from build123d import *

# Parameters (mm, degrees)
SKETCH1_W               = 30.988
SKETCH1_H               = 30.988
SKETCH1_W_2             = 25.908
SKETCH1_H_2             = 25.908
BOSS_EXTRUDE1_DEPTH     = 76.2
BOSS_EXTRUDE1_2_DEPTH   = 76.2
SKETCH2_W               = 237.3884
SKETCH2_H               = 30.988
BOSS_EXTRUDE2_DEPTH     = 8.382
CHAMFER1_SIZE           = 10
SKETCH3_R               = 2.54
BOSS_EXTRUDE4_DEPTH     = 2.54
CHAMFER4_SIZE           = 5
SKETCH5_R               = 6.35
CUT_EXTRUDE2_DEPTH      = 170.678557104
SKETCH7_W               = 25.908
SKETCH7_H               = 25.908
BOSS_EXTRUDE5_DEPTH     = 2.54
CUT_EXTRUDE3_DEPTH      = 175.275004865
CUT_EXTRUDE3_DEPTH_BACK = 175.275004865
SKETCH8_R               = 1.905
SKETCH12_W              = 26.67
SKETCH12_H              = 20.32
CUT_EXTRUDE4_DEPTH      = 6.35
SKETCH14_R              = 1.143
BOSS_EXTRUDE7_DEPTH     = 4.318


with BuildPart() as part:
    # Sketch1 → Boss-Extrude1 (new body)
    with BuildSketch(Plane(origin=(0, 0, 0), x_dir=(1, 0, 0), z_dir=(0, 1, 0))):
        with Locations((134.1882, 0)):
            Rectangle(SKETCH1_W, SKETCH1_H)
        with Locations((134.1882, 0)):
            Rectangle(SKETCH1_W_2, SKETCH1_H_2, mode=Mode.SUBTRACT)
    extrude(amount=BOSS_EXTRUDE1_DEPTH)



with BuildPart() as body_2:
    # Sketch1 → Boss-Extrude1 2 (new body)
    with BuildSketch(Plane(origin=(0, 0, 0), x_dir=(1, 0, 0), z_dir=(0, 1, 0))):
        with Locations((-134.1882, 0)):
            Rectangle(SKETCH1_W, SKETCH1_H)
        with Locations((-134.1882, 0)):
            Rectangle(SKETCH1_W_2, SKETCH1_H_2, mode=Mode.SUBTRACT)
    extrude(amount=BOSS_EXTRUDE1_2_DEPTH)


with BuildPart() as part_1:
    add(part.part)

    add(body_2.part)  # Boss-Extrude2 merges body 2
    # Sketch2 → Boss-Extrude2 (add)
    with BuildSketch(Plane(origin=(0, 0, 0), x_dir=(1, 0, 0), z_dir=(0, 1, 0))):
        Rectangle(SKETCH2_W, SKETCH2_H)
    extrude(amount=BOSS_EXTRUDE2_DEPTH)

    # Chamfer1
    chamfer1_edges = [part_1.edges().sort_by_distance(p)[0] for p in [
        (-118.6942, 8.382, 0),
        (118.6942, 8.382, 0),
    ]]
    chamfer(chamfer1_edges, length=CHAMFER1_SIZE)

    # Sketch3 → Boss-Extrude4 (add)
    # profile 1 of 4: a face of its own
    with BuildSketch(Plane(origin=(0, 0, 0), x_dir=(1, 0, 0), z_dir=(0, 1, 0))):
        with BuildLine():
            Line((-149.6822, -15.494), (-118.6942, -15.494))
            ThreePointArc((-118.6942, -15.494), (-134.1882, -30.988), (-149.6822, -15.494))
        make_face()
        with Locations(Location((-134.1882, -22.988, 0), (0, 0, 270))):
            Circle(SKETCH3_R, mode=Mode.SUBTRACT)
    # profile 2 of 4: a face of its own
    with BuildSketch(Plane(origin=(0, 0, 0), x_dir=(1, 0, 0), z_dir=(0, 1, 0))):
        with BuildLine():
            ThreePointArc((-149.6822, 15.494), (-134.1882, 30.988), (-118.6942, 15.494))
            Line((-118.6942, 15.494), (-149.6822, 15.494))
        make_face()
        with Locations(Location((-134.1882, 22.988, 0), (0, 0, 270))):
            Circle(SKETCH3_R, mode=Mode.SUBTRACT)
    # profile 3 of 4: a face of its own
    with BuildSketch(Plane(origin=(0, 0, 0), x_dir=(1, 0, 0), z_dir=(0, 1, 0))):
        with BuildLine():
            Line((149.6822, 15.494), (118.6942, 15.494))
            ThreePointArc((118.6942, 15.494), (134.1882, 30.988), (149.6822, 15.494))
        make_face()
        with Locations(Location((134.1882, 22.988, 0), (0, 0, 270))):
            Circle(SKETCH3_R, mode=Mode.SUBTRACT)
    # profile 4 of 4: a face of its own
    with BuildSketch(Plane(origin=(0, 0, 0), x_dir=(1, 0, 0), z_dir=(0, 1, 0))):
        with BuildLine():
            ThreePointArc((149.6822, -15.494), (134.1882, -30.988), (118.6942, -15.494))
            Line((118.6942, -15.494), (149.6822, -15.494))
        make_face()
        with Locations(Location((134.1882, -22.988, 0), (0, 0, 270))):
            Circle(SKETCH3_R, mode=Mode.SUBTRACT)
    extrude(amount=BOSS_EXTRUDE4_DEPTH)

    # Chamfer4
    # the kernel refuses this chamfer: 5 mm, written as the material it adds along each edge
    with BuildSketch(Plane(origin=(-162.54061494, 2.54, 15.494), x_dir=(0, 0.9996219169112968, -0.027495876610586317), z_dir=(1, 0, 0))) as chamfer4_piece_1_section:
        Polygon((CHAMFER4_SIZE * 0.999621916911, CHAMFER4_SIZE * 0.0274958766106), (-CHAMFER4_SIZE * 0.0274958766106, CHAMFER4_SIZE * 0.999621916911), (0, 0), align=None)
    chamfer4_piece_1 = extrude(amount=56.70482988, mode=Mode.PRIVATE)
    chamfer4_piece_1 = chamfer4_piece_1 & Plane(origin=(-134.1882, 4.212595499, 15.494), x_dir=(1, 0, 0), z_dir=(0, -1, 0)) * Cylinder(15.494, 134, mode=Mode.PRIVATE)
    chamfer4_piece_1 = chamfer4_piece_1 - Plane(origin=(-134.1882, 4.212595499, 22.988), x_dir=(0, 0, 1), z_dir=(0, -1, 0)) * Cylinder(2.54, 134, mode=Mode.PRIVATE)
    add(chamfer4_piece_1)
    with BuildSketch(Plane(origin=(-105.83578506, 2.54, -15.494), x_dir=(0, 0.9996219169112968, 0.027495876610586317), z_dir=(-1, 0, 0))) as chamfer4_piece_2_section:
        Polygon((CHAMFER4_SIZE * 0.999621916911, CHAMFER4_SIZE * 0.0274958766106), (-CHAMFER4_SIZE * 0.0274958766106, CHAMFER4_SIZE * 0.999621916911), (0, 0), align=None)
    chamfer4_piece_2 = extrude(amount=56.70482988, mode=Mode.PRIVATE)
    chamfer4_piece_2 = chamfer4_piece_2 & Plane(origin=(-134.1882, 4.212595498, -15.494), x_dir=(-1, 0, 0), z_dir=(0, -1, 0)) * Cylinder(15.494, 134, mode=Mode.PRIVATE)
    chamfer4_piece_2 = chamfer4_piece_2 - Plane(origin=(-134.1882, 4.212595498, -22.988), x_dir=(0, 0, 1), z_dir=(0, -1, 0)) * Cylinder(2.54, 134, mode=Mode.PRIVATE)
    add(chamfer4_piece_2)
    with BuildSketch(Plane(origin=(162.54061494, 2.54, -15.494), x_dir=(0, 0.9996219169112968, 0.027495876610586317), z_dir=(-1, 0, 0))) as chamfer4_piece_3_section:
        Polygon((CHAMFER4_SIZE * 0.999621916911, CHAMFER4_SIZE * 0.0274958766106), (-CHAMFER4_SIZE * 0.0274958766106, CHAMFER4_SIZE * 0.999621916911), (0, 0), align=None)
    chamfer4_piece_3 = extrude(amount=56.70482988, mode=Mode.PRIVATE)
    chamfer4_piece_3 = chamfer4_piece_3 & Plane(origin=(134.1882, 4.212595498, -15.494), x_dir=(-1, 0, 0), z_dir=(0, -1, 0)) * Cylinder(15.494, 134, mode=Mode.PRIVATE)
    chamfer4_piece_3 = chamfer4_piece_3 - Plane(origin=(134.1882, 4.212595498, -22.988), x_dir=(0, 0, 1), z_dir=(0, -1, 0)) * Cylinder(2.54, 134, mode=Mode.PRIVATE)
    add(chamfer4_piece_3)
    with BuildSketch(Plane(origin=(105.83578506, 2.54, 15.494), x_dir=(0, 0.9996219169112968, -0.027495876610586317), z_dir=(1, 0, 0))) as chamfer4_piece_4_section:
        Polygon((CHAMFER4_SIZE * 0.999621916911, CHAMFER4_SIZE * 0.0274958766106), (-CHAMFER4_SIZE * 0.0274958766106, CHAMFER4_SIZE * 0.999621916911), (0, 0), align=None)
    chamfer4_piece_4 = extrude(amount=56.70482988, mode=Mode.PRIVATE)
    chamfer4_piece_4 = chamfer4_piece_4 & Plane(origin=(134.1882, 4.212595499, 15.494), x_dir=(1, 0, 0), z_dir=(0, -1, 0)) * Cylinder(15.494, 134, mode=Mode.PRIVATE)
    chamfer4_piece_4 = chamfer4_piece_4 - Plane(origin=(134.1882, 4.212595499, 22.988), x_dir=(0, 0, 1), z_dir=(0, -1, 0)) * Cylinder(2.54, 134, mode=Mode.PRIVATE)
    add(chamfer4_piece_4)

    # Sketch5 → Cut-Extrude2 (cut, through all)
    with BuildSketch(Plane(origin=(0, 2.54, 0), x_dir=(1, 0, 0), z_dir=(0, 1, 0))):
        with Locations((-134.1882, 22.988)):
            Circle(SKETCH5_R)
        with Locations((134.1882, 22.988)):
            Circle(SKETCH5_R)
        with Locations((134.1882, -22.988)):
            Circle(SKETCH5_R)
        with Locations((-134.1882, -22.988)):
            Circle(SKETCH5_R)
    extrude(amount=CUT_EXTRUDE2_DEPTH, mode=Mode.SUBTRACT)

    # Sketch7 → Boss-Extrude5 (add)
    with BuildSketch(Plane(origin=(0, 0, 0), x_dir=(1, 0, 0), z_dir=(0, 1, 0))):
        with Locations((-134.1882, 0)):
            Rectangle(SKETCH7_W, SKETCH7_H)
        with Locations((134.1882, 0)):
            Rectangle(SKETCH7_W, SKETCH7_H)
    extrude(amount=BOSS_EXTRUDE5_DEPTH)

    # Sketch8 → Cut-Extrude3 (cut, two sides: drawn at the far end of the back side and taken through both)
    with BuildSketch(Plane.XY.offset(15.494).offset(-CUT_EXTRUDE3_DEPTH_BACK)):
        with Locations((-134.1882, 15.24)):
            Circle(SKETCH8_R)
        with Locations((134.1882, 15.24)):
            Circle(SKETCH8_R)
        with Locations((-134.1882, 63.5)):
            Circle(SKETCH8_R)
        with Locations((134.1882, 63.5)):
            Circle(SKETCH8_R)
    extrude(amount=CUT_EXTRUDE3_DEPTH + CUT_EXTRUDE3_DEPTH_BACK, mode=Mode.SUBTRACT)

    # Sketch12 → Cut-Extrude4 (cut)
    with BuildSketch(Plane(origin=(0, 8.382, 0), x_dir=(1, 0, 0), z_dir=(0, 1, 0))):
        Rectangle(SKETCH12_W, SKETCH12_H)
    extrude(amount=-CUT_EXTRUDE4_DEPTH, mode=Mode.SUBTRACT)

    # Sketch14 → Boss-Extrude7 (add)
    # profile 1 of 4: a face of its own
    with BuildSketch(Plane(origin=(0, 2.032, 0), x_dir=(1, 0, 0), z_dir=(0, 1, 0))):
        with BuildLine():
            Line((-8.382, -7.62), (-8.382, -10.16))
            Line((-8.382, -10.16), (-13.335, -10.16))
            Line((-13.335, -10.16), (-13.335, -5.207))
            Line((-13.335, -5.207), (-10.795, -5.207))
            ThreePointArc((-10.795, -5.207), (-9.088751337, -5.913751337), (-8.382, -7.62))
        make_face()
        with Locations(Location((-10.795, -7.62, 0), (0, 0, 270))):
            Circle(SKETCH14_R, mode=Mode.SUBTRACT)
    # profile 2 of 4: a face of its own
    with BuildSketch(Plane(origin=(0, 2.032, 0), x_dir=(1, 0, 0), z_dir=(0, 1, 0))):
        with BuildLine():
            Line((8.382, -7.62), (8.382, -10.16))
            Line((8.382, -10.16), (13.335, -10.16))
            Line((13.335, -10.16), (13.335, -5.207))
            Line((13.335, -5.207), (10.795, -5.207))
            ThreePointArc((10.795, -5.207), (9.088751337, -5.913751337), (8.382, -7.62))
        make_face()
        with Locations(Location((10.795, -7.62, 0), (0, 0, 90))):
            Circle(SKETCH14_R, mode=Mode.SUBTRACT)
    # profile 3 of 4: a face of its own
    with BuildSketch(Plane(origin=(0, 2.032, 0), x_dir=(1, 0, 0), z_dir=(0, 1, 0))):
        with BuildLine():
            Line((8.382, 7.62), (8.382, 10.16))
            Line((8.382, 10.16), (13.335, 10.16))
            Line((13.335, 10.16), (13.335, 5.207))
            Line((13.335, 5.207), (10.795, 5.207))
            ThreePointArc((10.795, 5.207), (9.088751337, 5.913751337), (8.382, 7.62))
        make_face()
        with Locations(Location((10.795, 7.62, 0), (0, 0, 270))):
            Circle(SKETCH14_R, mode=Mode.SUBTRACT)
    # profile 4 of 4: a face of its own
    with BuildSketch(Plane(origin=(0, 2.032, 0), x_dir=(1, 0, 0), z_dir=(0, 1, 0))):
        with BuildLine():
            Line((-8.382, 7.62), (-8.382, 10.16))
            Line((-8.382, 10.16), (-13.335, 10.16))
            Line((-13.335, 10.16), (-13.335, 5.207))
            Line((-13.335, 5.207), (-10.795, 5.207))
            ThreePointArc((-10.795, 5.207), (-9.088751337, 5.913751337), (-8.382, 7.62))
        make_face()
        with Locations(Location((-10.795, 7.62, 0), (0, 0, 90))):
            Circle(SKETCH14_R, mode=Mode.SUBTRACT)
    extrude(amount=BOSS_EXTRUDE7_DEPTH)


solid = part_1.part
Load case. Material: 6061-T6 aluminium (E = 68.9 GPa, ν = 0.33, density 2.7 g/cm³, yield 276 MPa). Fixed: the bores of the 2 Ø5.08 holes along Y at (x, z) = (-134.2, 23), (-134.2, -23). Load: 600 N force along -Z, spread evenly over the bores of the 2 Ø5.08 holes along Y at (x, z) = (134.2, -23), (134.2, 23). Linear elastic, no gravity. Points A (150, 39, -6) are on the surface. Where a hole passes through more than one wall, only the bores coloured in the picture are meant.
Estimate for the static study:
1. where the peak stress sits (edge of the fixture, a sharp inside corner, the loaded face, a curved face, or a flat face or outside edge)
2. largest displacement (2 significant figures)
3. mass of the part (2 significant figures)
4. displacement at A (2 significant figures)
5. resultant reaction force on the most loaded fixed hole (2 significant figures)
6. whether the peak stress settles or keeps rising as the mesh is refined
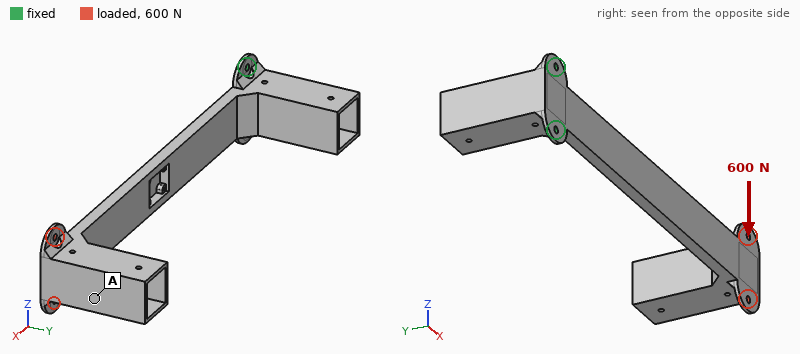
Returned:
edge of the fixture
3.1 mm
310 g
3.0 mm
3.6 kN
keeps rising
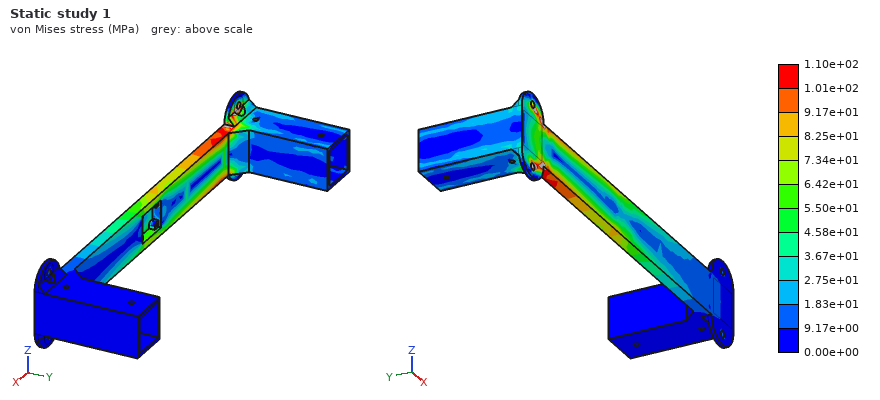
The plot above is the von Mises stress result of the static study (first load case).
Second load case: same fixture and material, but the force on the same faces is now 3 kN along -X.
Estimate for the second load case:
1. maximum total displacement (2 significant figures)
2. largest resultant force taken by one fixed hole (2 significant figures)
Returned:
3.3 mm
1.5 kN
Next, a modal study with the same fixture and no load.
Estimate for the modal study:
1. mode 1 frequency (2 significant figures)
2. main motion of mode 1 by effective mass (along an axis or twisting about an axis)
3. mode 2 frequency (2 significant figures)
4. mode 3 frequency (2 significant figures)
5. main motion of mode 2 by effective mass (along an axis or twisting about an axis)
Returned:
51 Hz
along Y
200 Hz
330 Hz
along Z
